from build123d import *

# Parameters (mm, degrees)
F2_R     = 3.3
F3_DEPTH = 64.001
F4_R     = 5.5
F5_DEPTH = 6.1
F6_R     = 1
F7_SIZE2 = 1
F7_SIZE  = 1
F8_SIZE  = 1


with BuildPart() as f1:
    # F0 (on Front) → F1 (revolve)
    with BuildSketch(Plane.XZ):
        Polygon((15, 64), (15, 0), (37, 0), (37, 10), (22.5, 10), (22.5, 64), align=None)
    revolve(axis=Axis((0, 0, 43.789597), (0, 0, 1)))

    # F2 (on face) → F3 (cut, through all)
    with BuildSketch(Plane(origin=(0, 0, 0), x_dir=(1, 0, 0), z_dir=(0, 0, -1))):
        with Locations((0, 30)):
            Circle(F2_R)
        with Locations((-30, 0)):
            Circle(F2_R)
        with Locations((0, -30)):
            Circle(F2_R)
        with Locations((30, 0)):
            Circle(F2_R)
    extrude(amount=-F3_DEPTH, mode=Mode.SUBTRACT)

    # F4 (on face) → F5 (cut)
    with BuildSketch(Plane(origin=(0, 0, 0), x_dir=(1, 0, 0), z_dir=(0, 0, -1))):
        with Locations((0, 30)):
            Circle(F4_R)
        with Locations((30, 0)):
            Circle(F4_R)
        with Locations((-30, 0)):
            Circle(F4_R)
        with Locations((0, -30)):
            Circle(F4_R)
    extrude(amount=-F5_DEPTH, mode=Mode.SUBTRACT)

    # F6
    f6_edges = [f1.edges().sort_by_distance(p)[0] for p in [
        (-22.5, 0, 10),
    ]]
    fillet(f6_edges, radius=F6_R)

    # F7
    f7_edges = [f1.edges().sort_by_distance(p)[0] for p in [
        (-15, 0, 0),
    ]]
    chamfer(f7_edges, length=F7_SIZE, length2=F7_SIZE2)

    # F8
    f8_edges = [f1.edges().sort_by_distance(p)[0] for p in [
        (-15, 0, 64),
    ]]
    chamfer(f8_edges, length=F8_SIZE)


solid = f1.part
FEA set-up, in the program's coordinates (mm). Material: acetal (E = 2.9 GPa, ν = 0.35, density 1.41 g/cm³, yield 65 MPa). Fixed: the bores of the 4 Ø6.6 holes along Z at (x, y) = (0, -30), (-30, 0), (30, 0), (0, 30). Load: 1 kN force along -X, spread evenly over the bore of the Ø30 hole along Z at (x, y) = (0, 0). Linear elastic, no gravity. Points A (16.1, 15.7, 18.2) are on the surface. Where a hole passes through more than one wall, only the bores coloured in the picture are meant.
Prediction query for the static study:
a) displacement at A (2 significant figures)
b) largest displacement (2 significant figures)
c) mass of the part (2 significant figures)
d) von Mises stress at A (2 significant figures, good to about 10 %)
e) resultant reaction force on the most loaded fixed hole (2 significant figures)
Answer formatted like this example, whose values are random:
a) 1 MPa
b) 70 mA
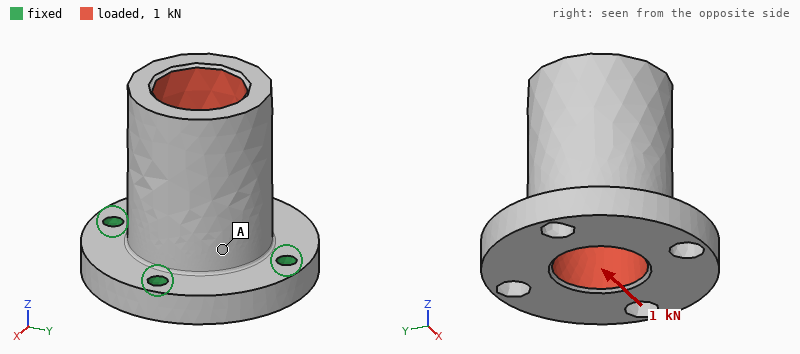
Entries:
a) 0.060 mm
b) 0.21 mm
c) 110 g
d) 1.9 MPa
e) 460 N
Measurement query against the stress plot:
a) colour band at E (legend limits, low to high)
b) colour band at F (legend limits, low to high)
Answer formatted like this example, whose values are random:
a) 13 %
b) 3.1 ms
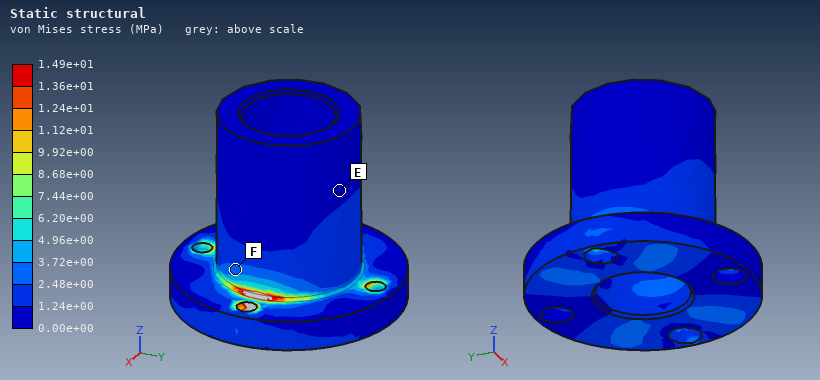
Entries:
a) 0.00e+00 to 1.24e+00 MPa
b) 2.48e+00 to 3.72e+00 MPa
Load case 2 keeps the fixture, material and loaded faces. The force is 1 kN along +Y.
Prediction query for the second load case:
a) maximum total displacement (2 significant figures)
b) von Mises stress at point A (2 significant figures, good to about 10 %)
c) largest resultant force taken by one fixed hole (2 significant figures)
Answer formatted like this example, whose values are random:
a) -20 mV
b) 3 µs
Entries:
a) 0.21 mm
b) 1.8 MPa
c) 460 N
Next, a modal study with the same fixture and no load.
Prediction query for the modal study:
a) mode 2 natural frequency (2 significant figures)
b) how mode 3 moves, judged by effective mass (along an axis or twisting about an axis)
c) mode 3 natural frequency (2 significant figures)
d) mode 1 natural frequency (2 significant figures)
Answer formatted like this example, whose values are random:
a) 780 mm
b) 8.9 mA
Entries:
a) 1400 Hz
b) along Z
c) 2800 Hz
d) 1400 Hz
